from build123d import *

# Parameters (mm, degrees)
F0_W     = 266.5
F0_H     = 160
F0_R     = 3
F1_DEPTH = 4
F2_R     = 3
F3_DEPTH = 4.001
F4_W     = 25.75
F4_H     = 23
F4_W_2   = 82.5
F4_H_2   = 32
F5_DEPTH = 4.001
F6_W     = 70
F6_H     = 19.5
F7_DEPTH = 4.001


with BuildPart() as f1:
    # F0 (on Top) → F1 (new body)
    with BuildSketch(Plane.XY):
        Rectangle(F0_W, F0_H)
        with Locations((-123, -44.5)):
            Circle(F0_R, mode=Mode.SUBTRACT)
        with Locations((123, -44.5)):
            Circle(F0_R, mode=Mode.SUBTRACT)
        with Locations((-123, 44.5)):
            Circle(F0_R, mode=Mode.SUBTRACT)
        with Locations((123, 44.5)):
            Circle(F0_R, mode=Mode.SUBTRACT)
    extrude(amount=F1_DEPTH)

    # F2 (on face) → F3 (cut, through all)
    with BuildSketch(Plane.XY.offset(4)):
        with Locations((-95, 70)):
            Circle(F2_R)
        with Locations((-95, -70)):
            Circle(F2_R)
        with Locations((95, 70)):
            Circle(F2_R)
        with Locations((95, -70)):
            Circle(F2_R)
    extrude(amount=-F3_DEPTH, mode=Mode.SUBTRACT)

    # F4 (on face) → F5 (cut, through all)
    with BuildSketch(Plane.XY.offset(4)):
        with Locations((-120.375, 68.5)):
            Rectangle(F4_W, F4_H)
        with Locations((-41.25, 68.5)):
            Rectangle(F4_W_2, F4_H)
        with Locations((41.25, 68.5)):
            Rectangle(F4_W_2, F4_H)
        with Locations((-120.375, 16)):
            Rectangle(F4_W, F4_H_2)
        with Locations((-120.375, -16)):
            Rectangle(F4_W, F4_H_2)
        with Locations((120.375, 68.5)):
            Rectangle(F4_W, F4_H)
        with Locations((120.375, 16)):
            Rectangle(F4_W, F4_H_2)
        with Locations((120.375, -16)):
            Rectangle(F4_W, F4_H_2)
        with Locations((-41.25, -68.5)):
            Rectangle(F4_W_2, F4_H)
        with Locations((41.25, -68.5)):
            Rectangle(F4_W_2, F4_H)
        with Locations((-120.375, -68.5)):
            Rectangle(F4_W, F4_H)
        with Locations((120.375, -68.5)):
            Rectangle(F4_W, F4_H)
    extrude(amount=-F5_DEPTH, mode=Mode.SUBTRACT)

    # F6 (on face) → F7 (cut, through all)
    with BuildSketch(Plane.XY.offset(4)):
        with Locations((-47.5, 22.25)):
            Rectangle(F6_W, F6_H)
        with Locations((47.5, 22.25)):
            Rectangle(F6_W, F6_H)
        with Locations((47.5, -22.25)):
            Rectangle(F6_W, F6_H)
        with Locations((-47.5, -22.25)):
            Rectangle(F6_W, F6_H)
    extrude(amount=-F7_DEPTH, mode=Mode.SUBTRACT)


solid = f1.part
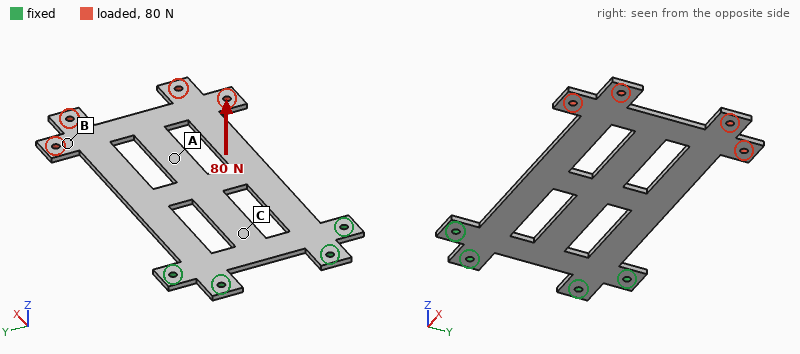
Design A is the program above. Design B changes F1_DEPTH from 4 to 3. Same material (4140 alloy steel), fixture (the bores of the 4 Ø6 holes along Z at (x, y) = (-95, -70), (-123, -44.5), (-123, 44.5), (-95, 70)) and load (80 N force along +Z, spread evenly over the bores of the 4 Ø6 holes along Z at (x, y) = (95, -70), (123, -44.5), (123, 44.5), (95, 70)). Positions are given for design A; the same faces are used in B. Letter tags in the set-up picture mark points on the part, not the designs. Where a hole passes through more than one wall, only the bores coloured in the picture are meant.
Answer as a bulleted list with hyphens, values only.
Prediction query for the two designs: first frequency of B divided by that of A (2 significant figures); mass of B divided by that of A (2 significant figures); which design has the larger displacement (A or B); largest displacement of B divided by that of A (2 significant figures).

- 0.75
- 0.75
- B
- 2.4
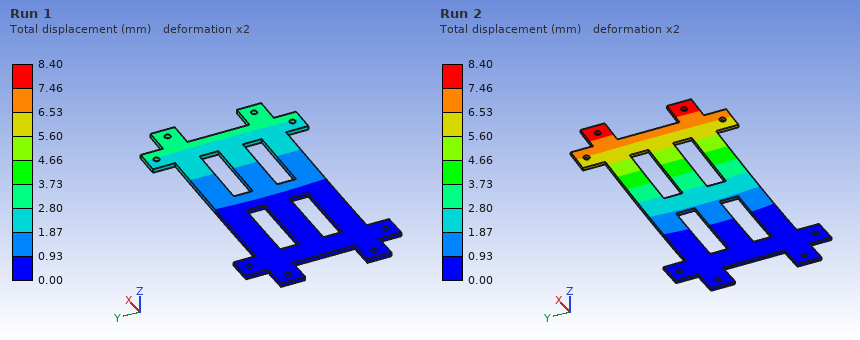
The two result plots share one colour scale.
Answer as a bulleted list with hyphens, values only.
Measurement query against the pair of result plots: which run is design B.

- Run 2
